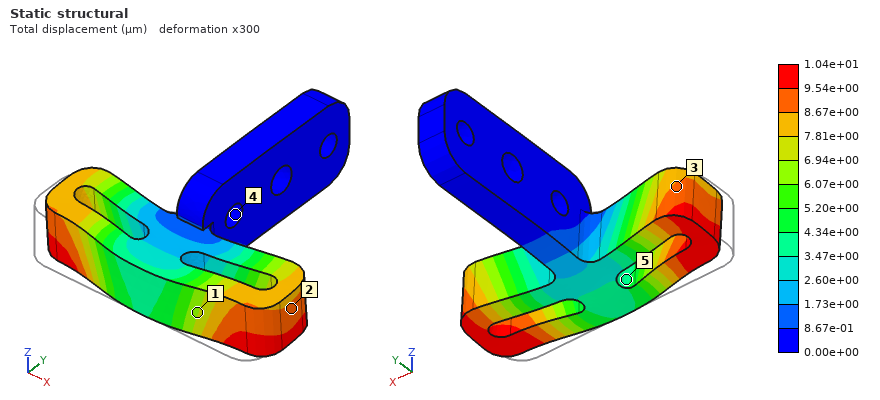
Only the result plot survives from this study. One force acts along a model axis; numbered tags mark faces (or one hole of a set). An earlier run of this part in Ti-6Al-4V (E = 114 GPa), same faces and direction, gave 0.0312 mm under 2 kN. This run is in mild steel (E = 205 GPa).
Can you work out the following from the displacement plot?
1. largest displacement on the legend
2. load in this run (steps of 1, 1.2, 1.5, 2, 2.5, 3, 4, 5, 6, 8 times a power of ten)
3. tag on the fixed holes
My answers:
1.04e+01 µm
1.2 kN
4
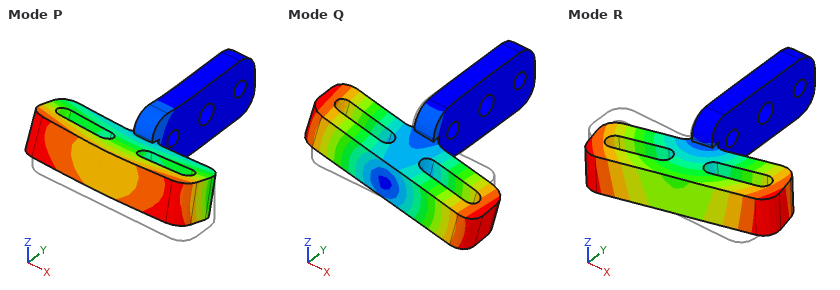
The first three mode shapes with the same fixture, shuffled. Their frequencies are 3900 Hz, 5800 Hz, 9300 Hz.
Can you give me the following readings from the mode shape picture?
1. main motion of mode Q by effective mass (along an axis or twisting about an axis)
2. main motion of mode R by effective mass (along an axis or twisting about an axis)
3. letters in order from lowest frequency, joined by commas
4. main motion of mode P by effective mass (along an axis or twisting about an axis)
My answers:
twisting about Y
along X
R, Q, P
along Z
